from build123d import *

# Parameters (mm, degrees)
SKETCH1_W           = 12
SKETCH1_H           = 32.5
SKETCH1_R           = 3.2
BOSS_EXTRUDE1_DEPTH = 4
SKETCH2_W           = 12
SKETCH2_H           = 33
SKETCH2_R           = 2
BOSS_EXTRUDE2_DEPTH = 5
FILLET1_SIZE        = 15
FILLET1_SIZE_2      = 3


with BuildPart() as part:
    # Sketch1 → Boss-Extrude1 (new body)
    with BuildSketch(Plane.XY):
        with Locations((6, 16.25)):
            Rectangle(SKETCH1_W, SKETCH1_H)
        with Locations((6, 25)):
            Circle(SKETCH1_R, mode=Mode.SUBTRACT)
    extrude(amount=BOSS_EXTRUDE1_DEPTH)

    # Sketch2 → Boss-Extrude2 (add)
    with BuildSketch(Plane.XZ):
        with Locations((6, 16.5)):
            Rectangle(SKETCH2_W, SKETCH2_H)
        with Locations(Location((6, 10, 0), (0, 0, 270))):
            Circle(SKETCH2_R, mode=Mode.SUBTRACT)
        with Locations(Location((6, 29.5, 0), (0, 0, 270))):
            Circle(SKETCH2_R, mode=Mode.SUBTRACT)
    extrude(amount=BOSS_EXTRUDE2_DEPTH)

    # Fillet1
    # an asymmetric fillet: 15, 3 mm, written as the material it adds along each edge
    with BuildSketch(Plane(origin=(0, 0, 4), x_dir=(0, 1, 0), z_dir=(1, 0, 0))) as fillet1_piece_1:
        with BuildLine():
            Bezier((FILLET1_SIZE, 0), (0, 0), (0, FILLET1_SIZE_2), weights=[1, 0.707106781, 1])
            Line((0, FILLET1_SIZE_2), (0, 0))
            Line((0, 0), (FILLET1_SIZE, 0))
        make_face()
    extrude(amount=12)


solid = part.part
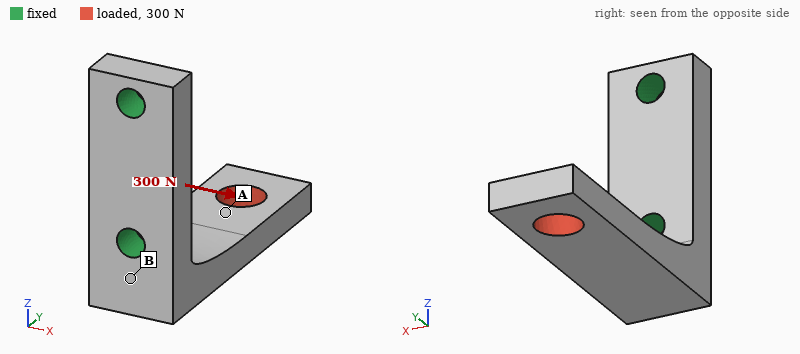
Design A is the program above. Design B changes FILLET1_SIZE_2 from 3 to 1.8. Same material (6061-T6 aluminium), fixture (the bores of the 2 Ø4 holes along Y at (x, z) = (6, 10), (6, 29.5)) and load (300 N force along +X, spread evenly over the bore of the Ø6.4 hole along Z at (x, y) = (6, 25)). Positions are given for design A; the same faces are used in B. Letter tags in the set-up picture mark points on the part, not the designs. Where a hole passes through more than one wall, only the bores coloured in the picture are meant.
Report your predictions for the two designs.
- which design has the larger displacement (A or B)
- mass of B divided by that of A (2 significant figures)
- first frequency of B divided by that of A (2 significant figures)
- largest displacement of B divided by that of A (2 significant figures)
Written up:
B
0.99
0.92
1.1
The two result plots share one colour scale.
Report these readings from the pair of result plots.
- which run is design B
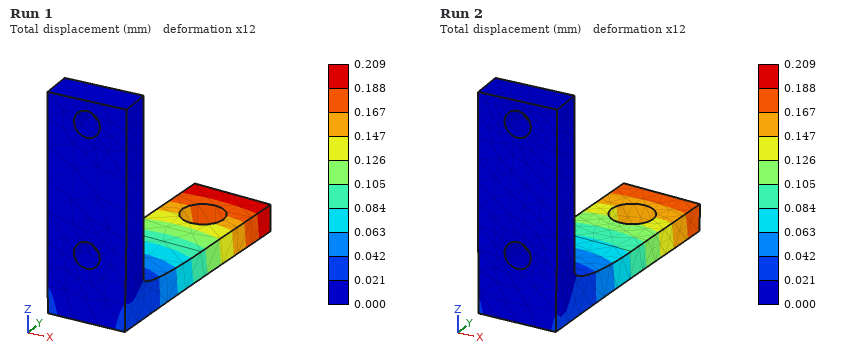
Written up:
Run 1
